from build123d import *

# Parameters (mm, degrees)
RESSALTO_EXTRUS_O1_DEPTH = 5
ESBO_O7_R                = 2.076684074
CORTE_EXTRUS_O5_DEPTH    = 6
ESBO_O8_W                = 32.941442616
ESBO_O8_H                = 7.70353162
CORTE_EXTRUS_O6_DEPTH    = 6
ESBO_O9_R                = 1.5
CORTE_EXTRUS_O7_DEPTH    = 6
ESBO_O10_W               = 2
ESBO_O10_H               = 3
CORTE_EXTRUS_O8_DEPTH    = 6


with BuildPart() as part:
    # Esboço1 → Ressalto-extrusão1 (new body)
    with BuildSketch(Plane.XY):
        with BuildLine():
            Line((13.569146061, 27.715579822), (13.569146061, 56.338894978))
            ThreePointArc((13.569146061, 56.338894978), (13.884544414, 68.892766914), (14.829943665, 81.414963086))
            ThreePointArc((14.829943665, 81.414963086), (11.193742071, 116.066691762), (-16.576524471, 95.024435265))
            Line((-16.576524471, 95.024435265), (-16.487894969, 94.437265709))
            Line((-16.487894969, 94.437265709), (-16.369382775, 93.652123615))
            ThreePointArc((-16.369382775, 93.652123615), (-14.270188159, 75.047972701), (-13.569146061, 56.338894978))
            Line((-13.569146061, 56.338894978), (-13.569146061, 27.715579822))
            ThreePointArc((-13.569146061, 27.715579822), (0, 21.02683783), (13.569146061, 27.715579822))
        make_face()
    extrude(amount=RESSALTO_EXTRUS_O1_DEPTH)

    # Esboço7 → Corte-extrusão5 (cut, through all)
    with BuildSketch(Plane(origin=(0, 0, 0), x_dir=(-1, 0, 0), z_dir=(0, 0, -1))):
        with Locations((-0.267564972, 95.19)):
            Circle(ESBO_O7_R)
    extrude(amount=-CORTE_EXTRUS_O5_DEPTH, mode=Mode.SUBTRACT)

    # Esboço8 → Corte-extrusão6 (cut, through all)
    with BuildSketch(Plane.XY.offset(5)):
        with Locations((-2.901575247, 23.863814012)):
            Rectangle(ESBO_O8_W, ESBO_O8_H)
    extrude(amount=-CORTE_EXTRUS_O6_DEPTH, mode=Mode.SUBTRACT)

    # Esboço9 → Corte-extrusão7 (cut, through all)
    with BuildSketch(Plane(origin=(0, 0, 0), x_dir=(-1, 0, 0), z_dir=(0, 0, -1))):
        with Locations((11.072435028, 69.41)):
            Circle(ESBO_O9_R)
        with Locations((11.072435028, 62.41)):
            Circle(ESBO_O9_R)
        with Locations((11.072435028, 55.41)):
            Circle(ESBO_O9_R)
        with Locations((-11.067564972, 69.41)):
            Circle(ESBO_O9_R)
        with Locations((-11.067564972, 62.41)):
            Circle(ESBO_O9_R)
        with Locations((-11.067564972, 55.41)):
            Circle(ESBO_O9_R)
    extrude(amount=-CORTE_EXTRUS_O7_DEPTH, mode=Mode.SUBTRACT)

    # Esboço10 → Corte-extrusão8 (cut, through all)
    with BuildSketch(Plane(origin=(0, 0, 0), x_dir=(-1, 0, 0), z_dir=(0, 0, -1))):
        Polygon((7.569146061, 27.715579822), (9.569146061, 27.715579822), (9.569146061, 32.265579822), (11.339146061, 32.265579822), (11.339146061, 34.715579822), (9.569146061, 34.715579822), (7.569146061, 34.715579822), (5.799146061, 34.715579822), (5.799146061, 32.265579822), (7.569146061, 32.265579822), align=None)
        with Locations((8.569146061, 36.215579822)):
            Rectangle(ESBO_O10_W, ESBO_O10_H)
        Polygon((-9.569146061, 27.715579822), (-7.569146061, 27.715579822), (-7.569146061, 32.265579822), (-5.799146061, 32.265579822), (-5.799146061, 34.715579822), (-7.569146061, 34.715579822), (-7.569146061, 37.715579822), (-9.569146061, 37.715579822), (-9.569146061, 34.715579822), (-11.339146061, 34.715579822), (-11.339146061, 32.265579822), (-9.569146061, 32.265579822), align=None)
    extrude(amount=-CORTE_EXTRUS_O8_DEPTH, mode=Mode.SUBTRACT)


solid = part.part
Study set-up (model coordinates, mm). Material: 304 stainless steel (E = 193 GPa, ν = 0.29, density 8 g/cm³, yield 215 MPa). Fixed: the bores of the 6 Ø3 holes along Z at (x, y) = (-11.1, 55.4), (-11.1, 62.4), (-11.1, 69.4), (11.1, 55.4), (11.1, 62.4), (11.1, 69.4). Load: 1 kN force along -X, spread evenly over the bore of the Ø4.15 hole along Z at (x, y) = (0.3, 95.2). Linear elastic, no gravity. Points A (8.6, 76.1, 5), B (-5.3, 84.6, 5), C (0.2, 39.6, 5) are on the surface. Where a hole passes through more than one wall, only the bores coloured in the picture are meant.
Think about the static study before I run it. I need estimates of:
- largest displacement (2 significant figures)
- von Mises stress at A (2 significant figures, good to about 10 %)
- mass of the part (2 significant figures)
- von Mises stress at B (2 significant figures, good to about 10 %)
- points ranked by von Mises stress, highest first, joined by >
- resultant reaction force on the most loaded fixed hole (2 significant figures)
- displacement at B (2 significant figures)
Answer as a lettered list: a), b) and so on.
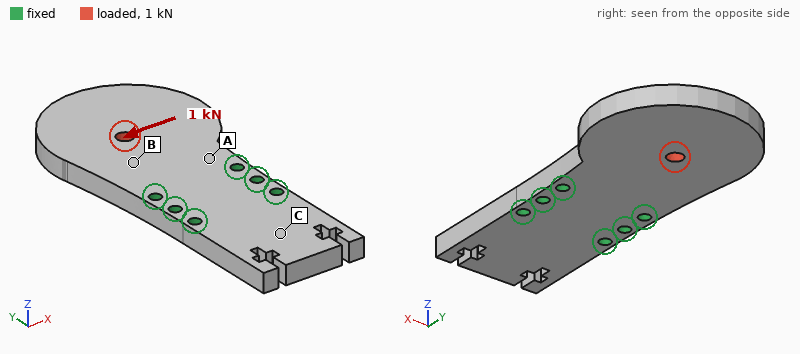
a) 9.7 µm
b) 22 MPa
c) 100 g
d) 17 MPa
e) A > B > C
f) 1.1 kN
g) 3.0 µm
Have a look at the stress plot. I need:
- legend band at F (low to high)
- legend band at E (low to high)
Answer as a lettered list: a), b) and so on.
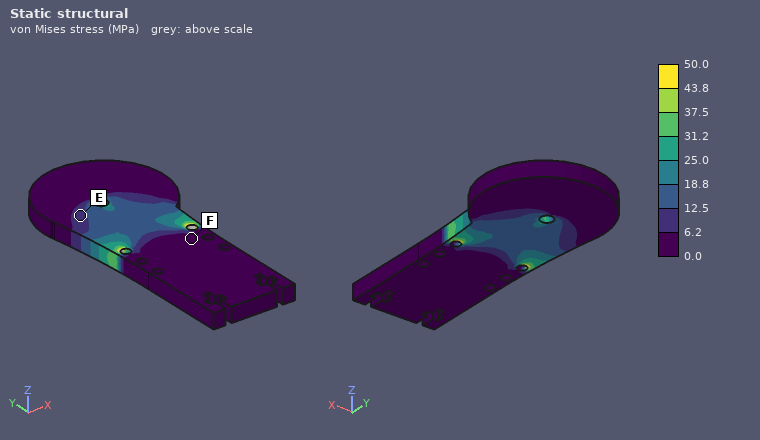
a) 0.0 to 6.2 MPa
b) 6.2 to 12.5 MPa
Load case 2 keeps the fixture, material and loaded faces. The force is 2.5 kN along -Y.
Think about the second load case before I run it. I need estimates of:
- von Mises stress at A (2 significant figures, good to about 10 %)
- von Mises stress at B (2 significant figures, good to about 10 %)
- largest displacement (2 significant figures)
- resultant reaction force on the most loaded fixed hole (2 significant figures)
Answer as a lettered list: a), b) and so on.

a) 20 MPa
b) 19 MPa
c) 3.6 µm
d) 960 N
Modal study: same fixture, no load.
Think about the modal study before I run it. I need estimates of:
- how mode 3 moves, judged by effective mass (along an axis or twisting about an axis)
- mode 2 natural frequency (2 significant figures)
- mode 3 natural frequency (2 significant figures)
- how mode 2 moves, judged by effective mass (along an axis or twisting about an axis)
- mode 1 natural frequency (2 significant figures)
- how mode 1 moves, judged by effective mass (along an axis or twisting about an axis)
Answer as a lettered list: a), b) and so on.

a) along Z
b) 5000 Hz
c) 5200 Hz
d) twisting about Y
e) 1700 Hz
f) along Z
